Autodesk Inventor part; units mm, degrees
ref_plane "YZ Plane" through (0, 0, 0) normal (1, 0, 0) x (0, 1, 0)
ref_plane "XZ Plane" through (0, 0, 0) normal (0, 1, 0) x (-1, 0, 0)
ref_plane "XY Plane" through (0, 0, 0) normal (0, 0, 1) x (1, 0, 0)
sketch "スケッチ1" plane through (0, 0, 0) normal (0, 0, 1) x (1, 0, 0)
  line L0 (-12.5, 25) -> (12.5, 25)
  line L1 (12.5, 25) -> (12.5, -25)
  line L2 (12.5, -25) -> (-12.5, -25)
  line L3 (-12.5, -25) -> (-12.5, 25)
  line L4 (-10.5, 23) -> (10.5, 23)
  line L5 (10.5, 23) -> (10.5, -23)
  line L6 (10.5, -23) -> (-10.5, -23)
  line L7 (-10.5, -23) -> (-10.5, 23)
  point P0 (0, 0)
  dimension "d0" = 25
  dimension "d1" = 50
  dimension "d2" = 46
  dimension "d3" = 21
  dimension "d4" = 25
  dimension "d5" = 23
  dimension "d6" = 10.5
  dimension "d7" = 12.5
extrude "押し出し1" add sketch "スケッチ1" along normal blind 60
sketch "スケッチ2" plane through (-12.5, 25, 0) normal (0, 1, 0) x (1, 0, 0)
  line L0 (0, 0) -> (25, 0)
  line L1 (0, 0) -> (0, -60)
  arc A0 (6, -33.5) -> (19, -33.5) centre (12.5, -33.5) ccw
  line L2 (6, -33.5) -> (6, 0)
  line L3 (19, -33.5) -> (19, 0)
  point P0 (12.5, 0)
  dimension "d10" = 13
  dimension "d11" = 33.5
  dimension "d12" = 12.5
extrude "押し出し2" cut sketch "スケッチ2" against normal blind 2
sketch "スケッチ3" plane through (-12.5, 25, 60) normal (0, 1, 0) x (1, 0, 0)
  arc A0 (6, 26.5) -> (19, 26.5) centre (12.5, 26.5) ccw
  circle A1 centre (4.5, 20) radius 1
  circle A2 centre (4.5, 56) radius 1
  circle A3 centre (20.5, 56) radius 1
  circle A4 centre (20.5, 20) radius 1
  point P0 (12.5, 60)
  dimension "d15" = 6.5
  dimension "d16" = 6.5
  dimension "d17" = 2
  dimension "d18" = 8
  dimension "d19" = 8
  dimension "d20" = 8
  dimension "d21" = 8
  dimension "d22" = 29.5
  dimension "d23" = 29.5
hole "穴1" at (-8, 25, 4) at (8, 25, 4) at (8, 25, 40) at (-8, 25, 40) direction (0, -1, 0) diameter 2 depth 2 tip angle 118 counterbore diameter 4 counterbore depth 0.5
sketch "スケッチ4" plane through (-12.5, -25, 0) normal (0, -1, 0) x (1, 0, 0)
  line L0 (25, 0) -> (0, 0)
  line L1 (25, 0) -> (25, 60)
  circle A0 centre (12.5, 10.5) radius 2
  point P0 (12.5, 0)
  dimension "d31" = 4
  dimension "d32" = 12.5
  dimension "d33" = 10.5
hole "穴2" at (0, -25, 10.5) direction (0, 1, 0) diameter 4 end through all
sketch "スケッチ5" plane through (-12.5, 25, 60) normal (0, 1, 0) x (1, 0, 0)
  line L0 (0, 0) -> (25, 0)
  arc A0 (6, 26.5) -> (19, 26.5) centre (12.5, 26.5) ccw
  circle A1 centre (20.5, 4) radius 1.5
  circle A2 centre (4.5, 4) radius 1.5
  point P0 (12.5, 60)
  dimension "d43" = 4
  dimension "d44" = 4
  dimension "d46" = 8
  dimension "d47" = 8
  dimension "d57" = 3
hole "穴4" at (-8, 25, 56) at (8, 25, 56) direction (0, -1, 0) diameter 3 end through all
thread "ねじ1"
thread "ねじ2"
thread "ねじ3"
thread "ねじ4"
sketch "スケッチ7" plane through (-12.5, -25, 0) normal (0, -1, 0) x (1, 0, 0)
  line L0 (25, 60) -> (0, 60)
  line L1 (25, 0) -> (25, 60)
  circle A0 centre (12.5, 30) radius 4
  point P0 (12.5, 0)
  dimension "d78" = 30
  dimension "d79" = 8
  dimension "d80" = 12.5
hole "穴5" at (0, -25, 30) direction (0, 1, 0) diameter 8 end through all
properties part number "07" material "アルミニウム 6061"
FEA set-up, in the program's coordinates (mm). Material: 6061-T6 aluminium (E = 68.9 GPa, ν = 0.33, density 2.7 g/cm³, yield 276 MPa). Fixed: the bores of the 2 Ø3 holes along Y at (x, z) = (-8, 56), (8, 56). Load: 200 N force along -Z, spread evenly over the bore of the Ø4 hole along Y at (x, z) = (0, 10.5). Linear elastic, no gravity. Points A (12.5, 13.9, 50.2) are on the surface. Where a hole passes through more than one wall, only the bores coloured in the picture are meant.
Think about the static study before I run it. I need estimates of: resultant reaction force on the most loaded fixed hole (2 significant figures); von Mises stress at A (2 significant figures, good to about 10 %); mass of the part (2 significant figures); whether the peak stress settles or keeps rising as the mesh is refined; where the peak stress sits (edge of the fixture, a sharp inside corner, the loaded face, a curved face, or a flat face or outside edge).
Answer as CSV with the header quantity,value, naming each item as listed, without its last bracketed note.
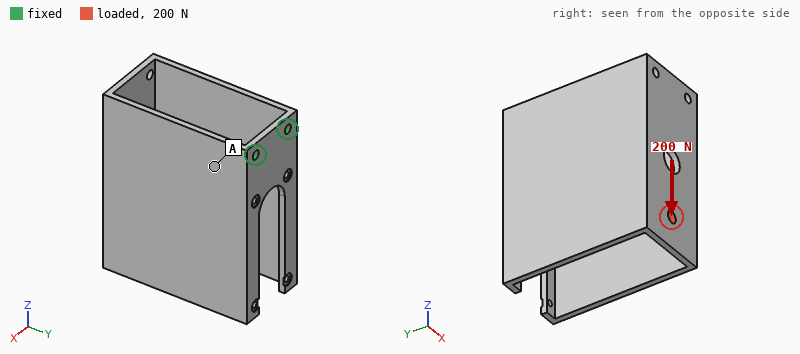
quantity,value
resultant reaction force on the most loaded fixed hole,100 N
von Mises stress at A,27 MPa
mass of the part,43 g
whether the peak stress settles or keeps rising as the mesh is refined,keeps rising
where the peak stress sits,edge of the fixture
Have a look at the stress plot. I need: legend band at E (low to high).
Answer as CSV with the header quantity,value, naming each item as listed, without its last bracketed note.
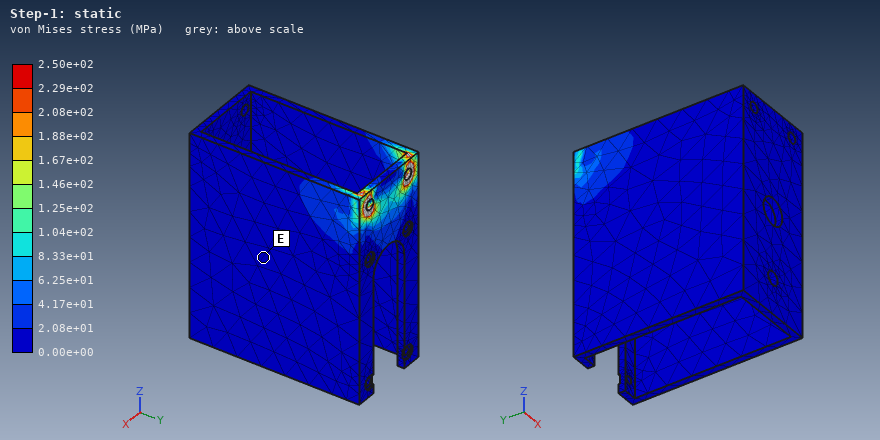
quantity,value
legend band at E,0.00e+00 to 2.08e+01 MPa
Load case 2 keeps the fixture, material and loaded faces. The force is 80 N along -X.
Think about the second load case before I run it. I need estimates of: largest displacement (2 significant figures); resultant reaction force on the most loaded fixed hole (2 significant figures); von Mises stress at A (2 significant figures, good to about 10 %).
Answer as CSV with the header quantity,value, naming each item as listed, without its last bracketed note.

quantity,value
largest displacement,0.33 mm
resultant reaction force on the most loaded fixed hole,250 N
von Mises stress at A,20 MPa
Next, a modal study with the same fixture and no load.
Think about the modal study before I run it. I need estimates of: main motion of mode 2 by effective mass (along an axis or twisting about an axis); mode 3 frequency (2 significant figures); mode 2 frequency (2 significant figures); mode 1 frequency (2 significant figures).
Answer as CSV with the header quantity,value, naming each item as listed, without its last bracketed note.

quantity,value
main motion of mode 2 by effective mass,along X
mode 3 frequency,1100 Hz
mode 2 frequency,580 Hz
mode 1 frequency,490 Hz
